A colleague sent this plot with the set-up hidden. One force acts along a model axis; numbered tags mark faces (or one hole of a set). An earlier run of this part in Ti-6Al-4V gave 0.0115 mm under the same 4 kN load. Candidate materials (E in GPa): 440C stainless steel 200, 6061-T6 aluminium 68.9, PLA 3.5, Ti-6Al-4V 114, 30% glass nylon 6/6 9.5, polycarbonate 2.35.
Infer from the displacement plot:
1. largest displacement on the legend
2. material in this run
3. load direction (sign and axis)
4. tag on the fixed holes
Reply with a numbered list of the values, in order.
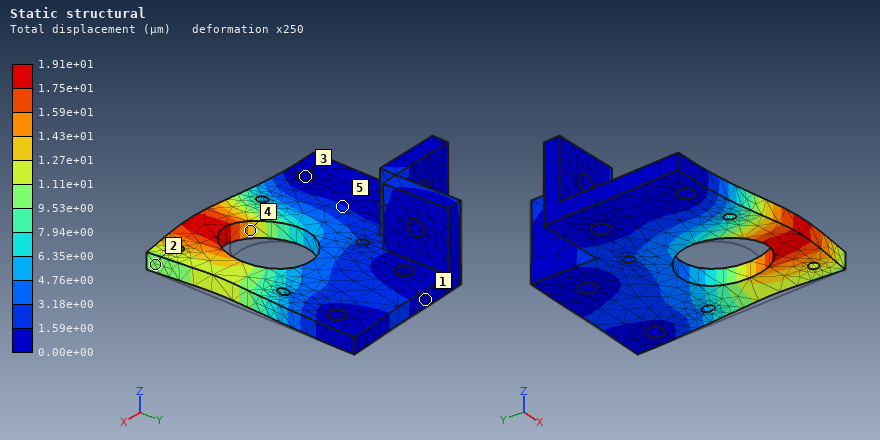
1. 1.91e+01 µm
2. 6061-T6 aluminium
3. -Y
4. 3
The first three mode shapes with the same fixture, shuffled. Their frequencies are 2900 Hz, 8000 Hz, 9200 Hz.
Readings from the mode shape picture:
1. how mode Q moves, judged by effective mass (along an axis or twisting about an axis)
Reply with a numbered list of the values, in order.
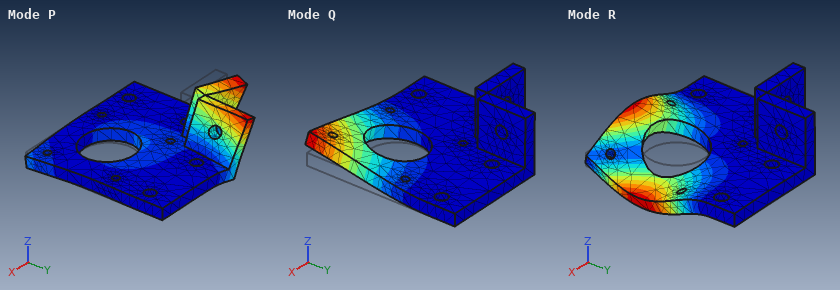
1. along Z
